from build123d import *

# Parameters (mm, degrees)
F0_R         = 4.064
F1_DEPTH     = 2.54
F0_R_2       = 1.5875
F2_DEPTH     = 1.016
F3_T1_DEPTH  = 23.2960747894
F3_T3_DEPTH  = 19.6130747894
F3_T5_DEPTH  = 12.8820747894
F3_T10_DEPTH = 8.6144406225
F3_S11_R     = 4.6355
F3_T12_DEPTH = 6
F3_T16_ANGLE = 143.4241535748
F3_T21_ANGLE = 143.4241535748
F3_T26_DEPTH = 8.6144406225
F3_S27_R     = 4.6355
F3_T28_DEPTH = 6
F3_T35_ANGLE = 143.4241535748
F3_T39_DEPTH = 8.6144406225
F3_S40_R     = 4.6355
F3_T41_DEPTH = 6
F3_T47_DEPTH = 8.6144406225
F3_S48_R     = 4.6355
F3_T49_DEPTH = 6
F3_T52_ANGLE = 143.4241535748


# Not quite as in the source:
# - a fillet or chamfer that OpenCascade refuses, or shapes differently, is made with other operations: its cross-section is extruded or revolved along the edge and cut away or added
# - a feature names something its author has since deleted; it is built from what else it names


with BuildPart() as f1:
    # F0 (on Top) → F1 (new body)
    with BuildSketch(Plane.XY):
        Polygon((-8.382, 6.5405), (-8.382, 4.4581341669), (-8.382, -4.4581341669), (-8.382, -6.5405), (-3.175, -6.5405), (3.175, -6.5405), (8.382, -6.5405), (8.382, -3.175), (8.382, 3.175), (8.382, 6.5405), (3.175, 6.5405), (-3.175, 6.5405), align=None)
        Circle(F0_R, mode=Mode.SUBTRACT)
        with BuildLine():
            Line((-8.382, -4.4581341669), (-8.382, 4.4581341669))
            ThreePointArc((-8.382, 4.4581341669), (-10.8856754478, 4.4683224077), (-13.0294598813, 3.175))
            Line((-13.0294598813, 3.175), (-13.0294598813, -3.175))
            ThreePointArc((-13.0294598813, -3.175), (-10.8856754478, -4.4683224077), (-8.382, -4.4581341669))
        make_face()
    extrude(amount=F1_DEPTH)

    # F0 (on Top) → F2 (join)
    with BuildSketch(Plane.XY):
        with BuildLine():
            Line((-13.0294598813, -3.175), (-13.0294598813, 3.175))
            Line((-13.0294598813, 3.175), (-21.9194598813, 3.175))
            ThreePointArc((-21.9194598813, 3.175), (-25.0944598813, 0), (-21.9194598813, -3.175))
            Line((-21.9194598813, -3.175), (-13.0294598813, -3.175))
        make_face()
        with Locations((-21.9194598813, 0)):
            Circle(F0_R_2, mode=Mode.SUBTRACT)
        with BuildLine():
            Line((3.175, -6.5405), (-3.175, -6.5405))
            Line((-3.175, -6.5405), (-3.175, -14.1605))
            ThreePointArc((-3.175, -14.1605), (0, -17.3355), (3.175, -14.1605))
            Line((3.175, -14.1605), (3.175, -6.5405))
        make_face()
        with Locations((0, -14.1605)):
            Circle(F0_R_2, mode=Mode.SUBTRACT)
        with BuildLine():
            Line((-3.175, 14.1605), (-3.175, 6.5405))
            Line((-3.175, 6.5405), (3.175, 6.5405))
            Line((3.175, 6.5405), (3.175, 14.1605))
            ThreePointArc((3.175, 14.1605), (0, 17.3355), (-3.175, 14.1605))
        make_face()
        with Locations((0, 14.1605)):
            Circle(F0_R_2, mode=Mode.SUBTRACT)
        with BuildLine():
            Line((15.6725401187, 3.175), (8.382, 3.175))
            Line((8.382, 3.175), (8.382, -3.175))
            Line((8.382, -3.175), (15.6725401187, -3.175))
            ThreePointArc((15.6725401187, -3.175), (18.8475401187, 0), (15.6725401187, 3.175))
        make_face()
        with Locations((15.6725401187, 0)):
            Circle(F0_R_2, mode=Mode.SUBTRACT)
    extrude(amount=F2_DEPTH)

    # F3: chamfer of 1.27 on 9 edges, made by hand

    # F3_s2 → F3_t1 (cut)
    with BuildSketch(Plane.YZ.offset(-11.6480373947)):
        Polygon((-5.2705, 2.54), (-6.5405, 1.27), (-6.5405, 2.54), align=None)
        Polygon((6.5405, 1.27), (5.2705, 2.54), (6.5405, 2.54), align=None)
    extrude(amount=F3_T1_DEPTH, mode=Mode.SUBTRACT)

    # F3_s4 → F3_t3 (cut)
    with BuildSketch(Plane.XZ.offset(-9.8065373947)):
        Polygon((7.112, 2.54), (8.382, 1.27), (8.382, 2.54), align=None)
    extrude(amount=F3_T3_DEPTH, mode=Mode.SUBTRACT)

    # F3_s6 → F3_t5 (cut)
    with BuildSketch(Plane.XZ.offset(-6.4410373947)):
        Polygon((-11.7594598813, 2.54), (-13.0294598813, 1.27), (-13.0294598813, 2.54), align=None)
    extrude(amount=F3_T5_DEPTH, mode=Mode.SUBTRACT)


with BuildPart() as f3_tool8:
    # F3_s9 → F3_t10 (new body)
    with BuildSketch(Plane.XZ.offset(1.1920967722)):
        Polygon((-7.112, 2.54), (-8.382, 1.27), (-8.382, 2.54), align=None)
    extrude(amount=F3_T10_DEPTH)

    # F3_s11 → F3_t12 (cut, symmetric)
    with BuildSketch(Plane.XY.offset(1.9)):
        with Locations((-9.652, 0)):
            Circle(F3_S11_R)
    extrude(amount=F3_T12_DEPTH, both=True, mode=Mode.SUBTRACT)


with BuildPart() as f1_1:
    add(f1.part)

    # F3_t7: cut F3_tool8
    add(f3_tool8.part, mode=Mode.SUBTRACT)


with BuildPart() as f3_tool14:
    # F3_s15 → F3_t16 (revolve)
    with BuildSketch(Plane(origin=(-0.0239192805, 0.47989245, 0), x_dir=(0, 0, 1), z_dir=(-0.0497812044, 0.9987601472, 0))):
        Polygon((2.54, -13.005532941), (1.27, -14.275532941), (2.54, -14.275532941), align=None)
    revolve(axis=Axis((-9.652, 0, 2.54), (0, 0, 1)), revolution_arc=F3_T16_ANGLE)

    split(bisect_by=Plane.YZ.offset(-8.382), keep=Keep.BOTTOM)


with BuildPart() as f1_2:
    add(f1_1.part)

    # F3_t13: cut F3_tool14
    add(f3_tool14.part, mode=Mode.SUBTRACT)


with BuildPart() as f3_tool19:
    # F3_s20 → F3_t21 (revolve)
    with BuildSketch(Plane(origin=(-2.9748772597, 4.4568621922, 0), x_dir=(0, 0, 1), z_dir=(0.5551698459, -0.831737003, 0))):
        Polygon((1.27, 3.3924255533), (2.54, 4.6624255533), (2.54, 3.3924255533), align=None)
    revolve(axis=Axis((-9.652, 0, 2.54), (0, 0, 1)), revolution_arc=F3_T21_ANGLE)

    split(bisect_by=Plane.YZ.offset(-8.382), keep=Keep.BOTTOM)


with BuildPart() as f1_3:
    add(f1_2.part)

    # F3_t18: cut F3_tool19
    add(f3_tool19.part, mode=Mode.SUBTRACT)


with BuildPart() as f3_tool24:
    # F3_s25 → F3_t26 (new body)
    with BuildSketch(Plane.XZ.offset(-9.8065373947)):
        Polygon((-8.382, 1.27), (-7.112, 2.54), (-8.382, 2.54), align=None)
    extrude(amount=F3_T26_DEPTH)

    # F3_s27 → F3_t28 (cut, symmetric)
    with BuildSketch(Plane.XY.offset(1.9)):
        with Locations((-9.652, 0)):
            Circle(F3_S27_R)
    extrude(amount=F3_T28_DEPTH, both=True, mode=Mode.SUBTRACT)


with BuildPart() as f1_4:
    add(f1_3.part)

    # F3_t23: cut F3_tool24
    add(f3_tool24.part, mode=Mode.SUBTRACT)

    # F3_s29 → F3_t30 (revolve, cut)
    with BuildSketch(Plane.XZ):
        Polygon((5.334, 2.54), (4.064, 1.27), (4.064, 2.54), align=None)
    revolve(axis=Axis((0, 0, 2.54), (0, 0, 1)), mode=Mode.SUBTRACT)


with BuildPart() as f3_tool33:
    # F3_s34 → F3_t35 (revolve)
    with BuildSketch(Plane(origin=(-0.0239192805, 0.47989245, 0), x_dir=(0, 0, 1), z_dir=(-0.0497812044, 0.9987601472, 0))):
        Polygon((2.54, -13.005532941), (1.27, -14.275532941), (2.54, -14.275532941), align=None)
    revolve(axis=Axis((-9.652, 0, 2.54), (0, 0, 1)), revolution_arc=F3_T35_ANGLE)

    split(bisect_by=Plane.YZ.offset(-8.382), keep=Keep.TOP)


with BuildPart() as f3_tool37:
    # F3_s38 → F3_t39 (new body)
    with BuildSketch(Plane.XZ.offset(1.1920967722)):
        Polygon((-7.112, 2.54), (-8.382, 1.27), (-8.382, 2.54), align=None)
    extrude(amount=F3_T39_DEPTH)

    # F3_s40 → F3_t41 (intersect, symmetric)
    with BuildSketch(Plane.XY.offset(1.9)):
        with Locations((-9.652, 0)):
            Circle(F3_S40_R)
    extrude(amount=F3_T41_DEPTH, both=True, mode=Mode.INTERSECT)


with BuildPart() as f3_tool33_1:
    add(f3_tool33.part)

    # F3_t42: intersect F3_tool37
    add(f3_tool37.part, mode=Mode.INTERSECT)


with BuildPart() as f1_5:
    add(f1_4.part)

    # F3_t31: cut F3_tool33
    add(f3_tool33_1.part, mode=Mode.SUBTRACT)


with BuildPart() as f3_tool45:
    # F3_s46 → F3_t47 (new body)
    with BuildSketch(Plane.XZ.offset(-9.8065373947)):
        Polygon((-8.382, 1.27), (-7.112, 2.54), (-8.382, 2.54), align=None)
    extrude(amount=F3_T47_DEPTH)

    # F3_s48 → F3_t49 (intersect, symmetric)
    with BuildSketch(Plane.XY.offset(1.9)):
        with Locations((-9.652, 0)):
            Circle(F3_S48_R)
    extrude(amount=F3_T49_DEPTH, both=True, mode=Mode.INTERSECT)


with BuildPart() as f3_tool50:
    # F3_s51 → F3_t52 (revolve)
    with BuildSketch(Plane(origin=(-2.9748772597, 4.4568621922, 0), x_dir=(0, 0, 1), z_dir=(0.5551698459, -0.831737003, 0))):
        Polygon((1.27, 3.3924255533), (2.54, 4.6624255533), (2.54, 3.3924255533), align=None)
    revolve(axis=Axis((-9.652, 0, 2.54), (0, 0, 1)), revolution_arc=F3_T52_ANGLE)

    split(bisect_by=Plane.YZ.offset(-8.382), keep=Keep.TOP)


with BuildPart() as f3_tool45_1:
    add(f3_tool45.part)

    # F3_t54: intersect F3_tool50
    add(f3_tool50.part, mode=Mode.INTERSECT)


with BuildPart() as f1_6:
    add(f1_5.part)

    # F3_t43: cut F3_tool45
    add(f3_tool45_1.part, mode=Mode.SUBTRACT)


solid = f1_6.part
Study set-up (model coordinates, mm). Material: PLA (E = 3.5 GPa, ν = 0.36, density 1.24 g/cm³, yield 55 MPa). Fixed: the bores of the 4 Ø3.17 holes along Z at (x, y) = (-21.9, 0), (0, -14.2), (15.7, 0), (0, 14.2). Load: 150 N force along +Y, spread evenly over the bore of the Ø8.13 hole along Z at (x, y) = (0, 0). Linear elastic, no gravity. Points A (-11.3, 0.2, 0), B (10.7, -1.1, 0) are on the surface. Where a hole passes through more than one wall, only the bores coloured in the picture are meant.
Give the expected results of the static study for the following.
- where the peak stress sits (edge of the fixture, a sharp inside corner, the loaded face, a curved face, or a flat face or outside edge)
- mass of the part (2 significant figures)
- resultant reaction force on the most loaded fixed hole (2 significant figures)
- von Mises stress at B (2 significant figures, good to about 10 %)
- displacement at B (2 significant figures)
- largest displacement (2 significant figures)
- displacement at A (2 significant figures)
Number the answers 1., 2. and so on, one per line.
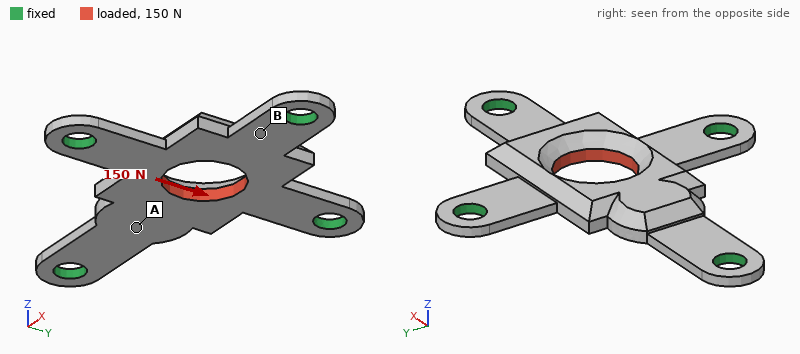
1. a flat face or outside edge
2. 0.85 g
3. 66 N
4. 4.5 MPa
5. 15 µm
6. 35 µm
7. 24 µm
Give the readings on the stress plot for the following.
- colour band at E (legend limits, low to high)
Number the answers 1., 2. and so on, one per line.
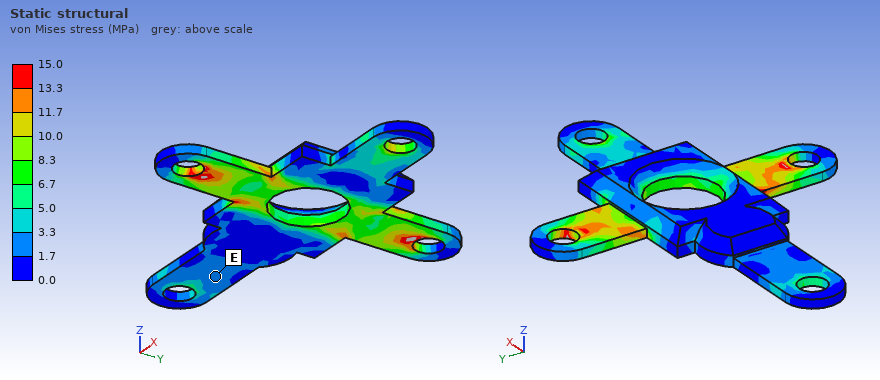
1. 1.7 to 3.3 MPa
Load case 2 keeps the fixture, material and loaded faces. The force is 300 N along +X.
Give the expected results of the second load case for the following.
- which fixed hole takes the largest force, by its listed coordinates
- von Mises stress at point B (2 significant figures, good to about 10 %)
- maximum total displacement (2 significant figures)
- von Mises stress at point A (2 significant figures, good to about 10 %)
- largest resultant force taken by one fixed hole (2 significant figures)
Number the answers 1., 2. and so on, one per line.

1. (15.7, 0)
2. 18 MPa
3. 78 µm
4. 14 MPa
5. 130 N
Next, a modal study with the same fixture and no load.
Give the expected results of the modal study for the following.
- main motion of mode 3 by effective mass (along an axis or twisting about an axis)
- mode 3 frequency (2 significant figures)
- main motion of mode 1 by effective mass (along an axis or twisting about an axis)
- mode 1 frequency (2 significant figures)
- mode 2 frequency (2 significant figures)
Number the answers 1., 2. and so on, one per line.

1. twisting about X
2. 5400 Hz
3. along Z
4. 2700 Hz
5. 4500 Hz
